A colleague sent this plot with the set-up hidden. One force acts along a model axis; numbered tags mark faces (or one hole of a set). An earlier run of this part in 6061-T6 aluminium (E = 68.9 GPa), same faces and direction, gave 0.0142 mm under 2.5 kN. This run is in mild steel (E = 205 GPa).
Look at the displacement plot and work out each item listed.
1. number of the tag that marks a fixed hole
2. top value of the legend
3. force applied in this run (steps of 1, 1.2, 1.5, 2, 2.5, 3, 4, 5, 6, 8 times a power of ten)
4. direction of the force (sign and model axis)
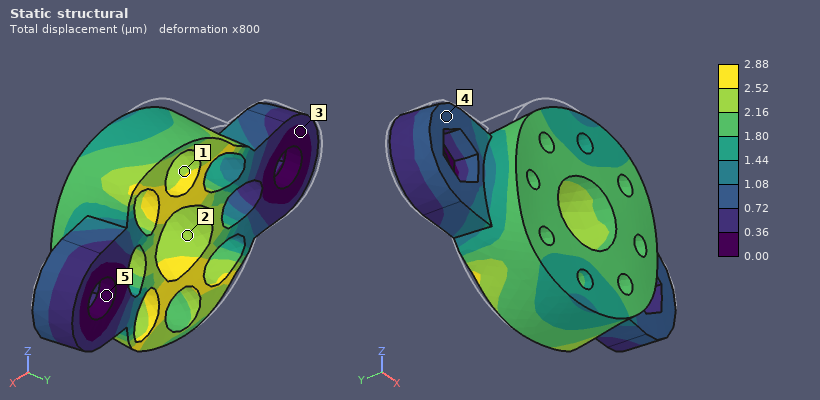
5
2.88 µm
1.5 kN
+X
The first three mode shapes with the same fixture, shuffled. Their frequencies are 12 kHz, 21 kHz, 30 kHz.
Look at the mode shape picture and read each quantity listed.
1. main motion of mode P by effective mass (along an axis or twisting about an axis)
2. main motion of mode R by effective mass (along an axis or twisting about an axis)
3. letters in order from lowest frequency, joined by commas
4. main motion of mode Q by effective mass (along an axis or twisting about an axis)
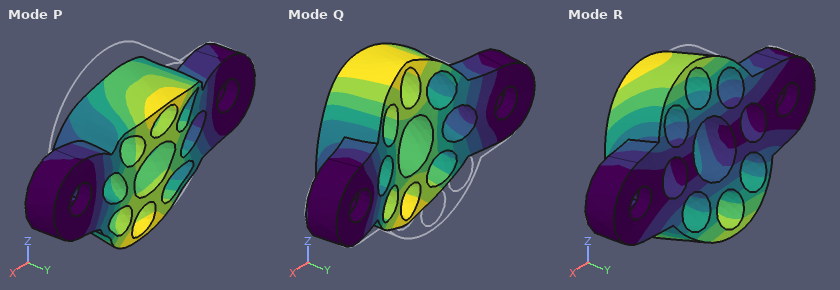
along Z
along Z
R, Q, P
along Y
